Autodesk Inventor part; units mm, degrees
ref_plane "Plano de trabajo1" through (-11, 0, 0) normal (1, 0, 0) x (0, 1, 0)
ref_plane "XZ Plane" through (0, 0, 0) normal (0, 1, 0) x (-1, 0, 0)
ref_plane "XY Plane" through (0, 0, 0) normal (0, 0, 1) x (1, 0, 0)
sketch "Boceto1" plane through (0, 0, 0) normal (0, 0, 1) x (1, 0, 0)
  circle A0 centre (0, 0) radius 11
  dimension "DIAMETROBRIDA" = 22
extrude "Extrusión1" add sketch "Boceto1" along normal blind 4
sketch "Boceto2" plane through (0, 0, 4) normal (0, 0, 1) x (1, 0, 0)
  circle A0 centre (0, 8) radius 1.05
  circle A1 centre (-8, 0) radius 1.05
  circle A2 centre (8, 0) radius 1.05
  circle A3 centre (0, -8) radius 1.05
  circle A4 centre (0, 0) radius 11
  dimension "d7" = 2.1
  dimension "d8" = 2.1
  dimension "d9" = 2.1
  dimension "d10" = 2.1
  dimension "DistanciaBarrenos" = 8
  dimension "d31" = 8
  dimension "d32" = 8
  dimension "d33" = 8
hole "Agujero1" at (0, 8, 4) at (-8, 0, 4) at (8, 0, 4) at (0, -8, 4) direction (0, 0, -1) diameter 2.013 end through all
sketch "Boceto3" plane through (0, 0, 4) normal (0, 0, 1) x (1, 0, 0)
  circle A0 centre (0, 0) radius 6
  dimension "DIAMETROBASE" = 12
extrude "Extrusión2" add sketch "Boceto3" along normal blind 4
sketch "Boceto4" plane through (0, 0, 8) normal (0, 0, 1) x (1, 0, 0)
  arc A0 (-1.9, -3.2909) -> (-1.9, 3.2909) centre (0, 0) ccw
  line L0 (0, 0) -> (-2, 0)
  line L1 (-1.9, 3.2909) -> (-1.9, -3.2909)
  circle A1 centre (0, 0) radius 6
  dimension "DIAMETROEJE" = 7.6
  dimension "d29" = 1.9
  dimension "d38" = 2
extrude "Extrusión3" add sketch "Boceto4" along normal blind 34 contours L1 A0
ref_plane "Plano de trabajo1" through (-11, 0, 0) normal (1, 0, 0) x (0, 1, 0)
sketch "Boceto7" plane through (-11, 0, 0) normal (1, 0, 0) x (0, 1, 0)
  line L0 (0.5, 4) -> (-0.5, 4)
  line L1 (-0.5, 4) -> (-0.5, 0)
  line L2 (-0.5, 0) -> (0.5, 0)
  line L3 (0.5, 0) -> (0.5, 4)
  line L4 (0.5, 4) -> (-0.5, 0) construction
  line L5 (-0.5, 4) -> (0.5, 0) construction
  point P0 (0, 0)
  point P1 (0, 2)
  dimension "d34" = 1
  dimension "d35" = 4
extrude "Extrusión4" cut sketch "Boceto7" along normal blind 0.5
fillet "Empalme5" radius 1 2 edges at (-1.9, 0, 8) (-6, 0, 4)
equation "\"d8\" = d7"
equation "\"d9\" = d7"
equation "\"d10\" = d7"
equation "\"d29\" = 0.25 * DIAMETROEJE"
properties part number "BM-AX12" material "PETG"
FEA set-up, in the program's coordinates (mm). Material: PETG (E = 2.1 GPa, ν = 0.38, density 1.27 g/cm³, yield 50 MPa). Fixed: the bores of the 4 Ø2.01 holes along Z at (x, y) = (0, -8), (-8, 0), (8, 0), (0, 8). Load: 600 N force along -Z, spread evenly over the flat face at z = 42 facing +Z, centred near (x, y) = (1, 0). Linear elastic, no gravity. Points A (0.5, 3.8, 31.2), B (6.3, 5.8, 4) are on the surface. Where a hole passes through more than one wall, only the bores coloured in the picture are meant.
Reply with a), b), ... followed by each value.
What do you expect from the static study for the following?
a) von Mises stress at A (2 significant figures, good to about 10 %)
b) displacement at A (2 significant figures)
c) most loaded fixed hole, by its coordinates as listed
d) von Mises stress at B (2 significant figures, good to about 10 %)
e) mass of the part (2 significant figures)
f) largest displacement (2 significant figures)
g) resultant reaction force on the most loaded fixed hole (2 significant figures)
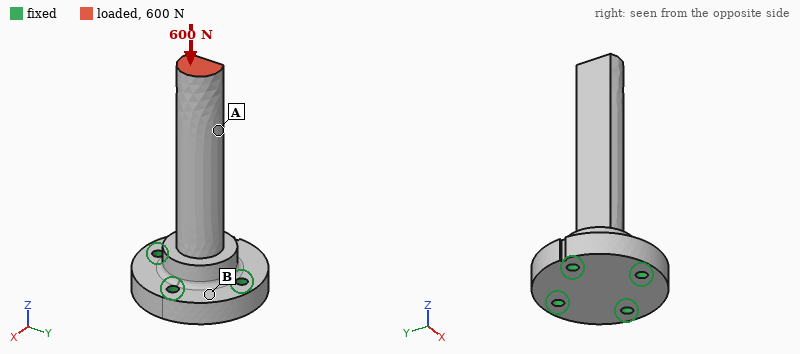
a) 16 MPa
b) 0.23 mm
c) (8, 0)
d) 3.3 MPa
e) 4.0 g
f) 0.32 mm
g) 180 N
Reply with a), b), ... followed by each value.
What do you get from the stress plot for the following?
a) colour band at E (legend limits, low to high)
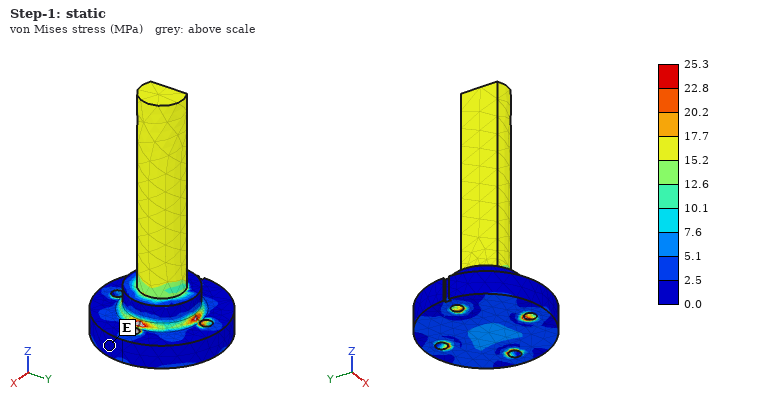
a) 0.0 to 2.5 MPa
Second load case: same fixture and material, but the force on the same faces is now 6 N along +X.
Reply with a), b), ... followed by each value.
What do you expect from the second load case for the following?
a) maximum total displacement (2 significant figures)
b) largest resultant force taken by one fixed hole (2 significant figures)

a) 0.53 mm
b) 16 N
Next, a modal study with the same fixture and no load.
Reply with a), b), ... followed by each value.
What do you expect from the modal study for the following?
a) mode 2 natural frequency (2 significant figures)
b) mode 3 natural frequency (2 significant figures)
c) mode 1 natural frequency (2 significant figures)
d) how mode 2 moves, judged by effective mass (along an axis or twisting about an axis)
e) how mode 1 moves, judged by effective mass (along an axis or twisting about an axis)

a) 1100 Hz
b) 4800 Hz
c) 850 Hz
d) along Y
e) along X
